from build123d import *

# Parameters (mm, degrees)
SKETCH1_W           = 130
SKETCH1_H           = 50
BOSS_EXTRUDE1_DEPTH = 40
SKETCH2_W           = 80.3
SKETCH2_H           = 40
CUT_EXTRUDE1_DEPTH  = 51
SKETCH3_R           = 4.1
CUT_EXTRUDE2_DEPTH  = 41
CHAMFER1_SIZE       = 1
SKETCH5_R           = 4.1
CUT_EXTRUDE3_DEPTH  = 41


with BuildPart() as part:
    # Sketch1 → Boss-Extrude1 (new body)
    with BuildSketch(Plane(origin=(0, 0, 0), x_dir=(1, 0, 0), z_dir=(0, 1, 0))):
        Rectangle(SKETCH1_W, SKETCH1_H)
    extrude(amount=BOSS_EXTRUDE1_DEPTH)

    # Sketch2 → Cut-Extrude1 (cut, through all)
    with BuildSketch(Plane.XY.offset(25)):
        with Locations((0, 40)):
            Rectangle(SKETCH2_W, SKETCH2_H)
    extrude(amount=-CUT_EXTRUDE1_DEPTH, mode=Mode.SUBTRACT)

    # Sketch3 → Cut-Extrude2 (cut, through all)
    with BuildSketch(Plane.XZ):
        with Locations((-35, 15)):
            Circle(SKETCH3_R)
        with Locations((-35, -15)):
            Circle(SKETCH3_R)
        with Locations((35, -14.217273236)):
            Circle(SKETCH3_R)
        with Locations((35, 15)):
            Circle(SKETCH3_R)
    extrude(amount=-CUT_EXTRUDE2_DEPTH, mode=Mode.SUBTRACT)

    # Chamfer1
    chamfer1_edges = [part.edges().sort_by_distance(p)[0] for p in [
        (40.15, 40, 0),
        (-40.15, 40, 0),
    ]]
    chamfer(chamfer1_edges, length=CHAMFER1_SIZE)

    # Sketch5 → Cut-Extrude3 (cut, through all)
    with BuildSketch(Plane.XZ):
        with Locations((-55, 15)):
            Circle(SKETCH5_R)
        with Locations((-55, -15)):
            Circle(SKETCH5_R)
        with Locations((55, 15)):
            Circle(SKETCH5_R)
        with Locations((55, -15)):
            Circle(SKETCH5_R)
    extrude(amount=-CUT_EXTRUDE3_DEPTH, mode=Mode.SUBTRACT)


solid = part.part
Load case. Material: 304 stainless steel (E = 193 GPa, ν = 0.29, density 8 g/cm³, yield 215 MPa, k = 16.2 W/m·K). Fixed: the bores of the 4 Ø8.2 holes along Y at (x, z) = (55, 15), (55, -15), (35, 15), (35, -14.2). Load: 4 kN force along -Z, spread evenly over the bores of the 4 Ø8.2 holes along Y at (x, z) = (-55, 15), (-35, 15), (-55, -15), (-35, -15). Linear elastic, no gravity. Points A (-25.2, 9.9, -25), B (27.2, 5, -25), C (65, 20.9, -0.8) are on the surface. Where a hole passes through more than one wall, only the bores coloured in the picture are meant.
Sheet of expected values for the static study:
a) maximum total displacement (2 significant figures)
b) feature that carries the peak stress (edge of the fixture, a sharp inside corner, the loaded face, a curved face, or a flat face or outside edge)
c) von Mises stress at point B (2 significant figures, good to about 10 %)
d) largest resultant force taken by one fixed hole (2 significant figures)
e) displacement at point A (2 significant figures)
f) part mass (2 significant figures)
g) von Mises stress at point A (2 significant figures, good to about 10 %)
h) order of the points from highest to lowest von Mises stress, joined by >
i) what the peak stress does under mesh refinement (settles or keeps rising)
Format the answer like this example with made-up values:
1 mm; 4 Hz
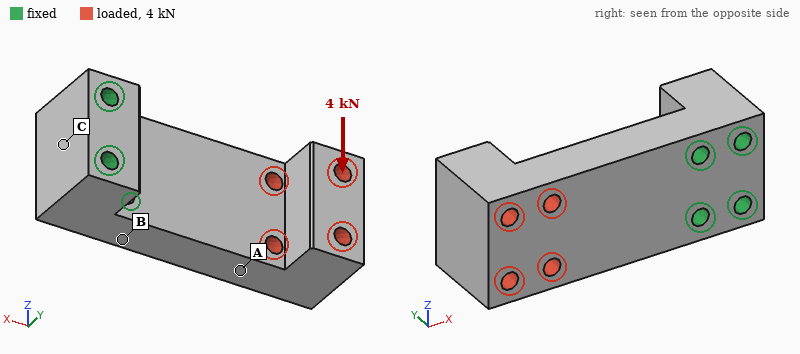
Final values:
40 µm; edge of the fixture; 29 MPa; 9.0 kN; 18 µm; 1.3 kg; 15 MPa; B > A > C; keeps rising
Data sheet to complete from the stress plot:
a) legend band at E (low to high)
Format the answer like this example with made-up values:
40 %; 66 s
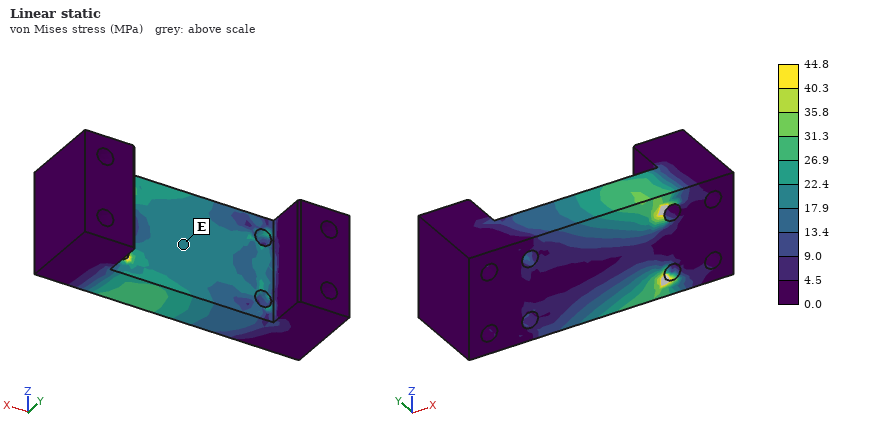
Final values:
17.9 to 22.4 MPa
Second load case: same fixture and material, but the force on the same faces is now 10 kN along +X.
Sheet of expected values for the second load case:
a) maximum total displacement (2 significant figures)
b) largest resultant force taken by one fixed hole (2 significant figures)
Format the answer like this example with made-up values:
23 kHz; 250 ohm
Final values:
61 µm; 4.4 kN
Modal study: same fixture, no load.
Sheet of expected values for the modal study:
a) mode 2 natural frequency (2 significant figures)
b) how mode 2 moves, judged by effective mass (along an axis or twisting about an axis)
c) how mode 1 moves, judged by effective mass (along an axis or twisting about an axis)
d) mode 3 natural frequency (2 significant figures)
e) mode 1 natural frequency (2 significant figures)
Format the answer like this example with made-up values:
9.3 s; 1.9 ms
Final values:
2600 Hz; along Z; along Y; 4200 Hz; 1200 Hz
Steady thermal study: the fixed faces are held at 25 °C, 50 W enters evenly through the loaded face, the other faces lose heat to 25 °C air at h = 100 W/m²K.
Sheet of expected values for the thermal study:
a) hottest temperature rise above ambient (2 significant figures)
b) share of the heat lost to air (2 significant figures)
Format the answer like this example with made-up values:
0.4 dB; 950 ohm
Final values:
47 K; 90 %
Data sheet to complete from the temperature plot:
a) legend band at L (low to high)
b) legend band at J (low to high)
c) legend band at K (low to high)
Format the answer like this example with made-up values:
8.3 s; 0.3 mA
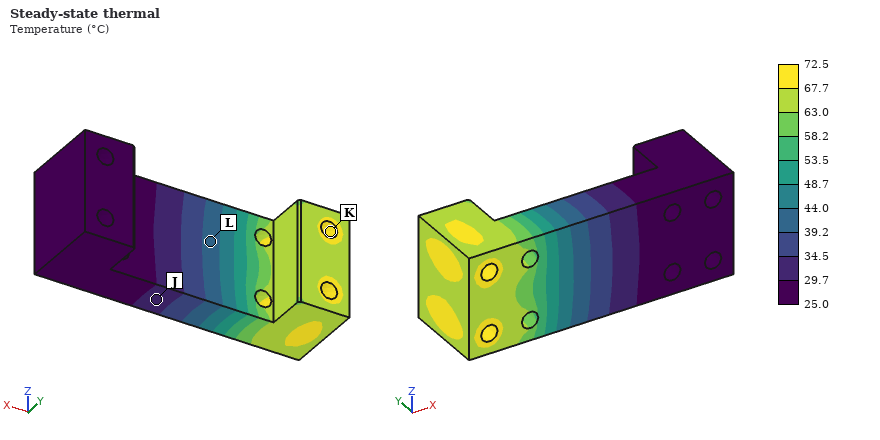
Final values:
39.2 to 44.0 °C; 29.7 to 34.5 °C; 67.7 to 72.5 °C
